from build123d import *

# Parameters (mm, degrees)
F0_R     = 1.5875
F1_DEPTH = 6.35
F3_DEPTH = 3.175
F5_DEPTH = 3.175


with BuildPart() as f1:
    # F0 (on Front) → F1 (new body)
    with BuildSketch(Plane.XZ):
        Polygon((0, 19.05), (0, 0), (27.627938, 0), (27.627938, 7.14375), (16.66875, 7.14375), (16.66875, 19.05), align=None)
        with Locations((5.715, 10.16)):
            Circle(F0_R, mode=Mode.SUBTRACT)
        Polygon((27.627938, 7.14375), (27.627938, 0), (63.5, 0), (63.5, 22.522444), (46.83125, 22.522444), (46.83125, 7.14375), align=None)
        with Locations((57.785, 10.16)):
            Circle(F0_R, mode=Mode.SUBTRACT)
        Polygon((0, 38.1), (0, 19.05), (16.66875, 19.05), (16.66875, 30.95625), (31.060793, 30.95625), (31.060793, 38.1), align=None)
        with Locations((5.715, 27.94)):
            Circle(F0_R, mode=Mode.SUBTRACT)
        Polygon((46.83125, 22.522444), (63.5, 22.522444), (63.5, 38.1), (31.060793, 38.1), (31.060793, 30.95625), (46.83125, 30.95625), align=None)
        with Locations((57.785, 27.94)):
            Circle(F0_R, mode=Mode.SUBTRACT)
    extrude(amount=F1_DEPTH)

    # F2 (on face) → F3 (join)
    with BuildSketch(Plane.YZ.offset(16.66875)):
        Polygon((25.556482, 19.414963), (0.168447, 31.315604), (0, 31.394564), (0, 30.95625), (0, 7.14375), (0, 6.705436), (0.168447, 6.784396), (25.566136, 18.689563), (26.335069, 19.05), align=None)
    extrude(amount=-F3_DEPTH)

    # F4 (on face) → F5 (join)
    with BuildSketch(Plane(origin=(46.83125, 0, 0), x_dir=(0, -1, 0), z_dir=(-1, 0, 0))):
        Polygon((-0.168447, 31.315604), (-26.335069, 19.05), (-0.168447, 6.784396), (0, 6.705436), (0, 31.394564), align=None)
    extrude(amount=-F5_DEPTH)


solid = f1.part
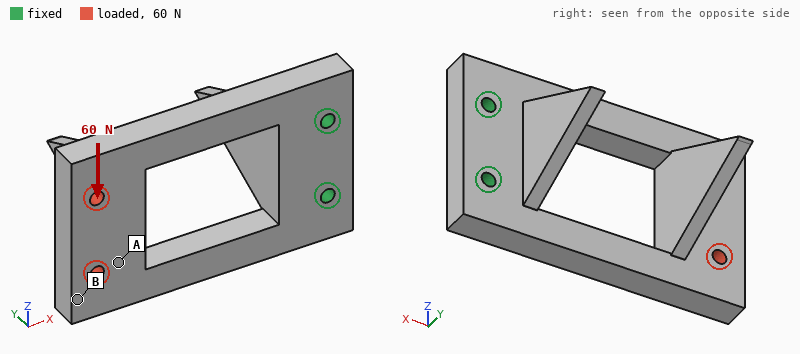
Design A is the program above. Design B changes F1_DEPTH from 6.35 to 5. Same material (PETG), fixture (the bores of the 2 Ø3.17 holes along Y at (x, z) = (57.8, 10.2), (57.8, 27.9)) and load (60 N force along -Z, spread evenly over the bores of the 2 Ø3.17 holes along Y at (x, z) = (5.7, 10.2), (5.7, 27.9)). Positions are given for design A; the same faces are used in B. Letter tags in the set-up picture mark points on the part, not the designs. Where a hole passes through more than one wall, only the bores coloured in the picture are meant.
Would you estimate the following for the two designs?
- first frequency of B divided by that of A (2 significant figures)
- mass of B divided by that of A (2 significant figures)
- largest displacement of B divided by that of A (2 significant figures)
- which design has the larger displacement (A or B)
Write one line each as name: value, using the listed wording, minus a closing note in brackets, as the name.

first frequency of B divided by that of A: 0.79
mass of B divided by that of A: 0.82
largest displacement of B divided by that of A: 1.3
which design has the larger displacement: B
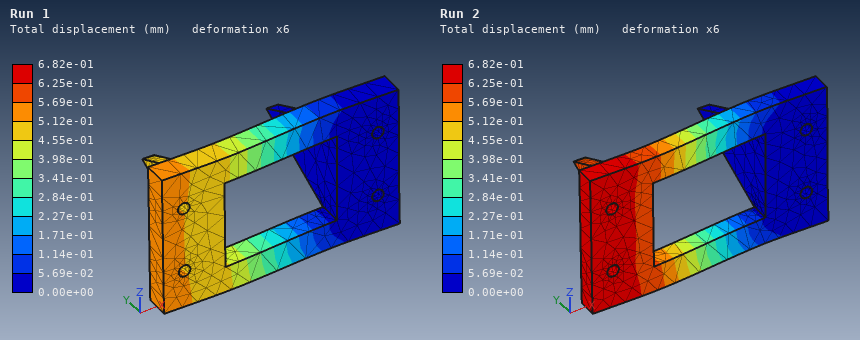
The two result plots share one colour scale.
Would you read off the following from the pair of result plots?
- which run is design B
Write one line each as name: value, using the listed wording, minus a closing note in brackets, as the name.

which run is design B: Run 2
